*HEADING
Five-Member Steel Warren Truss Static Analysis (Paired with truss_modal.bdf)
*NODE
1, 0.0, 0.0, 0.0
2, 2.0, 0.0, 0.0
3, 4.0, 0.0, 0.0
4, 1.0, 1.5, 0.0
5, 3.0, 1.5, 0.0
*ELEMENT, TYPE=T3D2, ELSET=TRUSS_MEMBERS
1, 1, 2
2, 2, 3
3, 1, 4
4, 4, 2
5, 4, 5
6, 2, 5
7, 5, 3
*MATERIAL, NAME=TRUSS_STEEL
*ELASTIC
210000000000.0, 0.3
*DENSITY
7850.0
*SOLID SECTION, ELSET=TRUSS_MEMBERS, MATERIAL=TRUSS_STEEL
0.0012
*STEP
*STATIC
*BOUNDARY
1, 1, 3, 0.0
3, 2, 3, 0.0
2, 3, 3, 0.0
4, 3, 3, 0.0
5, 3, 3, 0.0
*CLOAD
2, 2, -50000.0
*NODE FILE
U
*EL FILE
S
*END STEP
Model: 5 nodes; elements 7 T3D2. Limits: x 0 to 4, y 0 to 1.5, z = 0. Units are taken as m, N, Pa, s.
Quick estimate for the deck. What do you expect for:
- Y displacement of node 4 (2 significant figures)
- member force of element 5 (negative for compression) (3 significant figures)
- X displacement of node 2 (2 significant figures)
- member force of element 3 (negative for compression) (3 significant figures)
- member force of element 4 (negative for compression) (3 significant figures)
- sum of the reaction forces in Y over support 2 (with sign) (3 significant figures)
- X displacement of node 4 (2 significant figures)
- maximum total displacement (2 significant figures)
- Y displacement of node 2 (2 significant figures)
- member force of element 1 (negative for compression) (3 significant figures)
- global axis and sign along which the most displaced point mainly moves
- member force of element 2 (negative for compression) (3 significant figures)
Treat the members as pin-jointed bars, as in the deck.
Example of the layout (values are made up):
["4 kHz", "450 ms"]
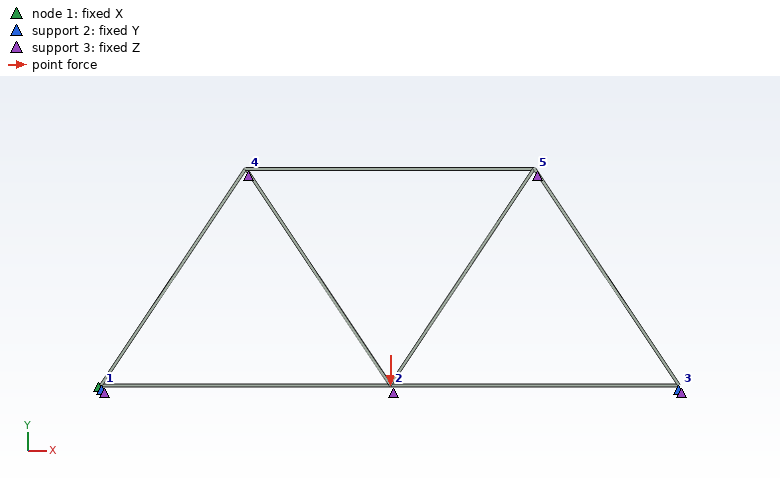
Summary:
["-4.3e-04 m", "-33300 N", "1.3e-04 m", "-30000 N", "30000 N", "50000 N", "2.6e-04 m", "7.9e-04 m", "-7.8e-04 m", "16700 N", "-Y", "16700 N"]
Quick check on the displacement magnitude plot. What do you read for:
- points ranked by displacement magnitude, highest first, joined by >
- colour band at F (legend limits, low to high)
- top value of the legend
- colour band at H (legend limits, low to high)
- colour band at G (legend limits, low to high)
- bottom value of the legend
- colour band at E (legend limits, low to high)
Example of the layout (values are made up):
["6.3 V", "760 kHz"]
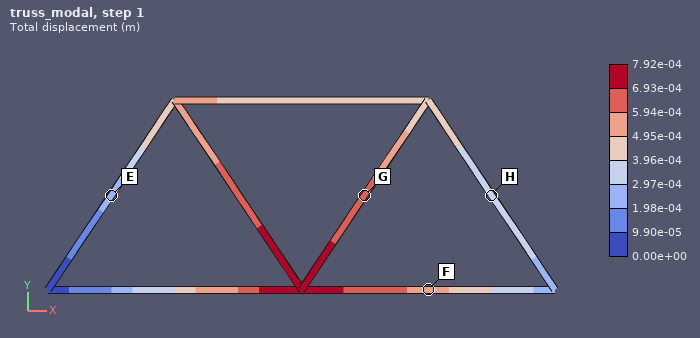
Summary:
["G > F > H > E", "4.95e-04 to 5.94e-04 m", "7.92e-04 m", "2.97e-04 to 3.96e-04 m", "5.94e-04 to 6.93e-04 m", "0.00e+00 m", "1.98e-04 to 2.97e-04 m"]
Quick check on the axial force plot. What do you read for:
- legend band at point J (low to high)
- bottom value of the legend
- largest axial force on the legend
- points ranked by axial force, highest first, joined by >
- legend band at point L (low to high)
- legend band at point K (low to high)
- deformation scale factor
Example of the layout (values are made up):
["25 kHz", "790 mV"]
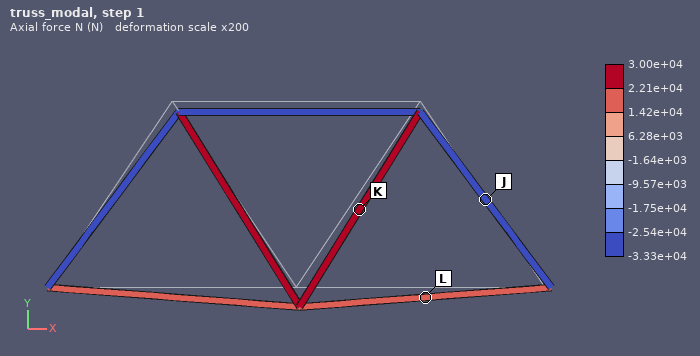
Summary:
["-3.33e+04 to -2.54e+04 N", "-3.33e+04 N", "3.00e+04 N", "K > L > J", "1.42e+04 to 2.21e+04 N", "2.21e+04 to 3.00e+04 N", "200"]
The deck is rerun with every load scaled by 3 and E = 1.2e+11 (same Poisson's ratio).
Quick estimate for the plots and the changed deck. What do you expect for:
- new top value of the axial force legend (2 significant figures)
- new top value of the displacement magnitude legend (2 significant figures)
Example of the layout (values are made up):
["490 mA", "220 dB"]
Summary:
["90000 N", "0.0042 m"]
